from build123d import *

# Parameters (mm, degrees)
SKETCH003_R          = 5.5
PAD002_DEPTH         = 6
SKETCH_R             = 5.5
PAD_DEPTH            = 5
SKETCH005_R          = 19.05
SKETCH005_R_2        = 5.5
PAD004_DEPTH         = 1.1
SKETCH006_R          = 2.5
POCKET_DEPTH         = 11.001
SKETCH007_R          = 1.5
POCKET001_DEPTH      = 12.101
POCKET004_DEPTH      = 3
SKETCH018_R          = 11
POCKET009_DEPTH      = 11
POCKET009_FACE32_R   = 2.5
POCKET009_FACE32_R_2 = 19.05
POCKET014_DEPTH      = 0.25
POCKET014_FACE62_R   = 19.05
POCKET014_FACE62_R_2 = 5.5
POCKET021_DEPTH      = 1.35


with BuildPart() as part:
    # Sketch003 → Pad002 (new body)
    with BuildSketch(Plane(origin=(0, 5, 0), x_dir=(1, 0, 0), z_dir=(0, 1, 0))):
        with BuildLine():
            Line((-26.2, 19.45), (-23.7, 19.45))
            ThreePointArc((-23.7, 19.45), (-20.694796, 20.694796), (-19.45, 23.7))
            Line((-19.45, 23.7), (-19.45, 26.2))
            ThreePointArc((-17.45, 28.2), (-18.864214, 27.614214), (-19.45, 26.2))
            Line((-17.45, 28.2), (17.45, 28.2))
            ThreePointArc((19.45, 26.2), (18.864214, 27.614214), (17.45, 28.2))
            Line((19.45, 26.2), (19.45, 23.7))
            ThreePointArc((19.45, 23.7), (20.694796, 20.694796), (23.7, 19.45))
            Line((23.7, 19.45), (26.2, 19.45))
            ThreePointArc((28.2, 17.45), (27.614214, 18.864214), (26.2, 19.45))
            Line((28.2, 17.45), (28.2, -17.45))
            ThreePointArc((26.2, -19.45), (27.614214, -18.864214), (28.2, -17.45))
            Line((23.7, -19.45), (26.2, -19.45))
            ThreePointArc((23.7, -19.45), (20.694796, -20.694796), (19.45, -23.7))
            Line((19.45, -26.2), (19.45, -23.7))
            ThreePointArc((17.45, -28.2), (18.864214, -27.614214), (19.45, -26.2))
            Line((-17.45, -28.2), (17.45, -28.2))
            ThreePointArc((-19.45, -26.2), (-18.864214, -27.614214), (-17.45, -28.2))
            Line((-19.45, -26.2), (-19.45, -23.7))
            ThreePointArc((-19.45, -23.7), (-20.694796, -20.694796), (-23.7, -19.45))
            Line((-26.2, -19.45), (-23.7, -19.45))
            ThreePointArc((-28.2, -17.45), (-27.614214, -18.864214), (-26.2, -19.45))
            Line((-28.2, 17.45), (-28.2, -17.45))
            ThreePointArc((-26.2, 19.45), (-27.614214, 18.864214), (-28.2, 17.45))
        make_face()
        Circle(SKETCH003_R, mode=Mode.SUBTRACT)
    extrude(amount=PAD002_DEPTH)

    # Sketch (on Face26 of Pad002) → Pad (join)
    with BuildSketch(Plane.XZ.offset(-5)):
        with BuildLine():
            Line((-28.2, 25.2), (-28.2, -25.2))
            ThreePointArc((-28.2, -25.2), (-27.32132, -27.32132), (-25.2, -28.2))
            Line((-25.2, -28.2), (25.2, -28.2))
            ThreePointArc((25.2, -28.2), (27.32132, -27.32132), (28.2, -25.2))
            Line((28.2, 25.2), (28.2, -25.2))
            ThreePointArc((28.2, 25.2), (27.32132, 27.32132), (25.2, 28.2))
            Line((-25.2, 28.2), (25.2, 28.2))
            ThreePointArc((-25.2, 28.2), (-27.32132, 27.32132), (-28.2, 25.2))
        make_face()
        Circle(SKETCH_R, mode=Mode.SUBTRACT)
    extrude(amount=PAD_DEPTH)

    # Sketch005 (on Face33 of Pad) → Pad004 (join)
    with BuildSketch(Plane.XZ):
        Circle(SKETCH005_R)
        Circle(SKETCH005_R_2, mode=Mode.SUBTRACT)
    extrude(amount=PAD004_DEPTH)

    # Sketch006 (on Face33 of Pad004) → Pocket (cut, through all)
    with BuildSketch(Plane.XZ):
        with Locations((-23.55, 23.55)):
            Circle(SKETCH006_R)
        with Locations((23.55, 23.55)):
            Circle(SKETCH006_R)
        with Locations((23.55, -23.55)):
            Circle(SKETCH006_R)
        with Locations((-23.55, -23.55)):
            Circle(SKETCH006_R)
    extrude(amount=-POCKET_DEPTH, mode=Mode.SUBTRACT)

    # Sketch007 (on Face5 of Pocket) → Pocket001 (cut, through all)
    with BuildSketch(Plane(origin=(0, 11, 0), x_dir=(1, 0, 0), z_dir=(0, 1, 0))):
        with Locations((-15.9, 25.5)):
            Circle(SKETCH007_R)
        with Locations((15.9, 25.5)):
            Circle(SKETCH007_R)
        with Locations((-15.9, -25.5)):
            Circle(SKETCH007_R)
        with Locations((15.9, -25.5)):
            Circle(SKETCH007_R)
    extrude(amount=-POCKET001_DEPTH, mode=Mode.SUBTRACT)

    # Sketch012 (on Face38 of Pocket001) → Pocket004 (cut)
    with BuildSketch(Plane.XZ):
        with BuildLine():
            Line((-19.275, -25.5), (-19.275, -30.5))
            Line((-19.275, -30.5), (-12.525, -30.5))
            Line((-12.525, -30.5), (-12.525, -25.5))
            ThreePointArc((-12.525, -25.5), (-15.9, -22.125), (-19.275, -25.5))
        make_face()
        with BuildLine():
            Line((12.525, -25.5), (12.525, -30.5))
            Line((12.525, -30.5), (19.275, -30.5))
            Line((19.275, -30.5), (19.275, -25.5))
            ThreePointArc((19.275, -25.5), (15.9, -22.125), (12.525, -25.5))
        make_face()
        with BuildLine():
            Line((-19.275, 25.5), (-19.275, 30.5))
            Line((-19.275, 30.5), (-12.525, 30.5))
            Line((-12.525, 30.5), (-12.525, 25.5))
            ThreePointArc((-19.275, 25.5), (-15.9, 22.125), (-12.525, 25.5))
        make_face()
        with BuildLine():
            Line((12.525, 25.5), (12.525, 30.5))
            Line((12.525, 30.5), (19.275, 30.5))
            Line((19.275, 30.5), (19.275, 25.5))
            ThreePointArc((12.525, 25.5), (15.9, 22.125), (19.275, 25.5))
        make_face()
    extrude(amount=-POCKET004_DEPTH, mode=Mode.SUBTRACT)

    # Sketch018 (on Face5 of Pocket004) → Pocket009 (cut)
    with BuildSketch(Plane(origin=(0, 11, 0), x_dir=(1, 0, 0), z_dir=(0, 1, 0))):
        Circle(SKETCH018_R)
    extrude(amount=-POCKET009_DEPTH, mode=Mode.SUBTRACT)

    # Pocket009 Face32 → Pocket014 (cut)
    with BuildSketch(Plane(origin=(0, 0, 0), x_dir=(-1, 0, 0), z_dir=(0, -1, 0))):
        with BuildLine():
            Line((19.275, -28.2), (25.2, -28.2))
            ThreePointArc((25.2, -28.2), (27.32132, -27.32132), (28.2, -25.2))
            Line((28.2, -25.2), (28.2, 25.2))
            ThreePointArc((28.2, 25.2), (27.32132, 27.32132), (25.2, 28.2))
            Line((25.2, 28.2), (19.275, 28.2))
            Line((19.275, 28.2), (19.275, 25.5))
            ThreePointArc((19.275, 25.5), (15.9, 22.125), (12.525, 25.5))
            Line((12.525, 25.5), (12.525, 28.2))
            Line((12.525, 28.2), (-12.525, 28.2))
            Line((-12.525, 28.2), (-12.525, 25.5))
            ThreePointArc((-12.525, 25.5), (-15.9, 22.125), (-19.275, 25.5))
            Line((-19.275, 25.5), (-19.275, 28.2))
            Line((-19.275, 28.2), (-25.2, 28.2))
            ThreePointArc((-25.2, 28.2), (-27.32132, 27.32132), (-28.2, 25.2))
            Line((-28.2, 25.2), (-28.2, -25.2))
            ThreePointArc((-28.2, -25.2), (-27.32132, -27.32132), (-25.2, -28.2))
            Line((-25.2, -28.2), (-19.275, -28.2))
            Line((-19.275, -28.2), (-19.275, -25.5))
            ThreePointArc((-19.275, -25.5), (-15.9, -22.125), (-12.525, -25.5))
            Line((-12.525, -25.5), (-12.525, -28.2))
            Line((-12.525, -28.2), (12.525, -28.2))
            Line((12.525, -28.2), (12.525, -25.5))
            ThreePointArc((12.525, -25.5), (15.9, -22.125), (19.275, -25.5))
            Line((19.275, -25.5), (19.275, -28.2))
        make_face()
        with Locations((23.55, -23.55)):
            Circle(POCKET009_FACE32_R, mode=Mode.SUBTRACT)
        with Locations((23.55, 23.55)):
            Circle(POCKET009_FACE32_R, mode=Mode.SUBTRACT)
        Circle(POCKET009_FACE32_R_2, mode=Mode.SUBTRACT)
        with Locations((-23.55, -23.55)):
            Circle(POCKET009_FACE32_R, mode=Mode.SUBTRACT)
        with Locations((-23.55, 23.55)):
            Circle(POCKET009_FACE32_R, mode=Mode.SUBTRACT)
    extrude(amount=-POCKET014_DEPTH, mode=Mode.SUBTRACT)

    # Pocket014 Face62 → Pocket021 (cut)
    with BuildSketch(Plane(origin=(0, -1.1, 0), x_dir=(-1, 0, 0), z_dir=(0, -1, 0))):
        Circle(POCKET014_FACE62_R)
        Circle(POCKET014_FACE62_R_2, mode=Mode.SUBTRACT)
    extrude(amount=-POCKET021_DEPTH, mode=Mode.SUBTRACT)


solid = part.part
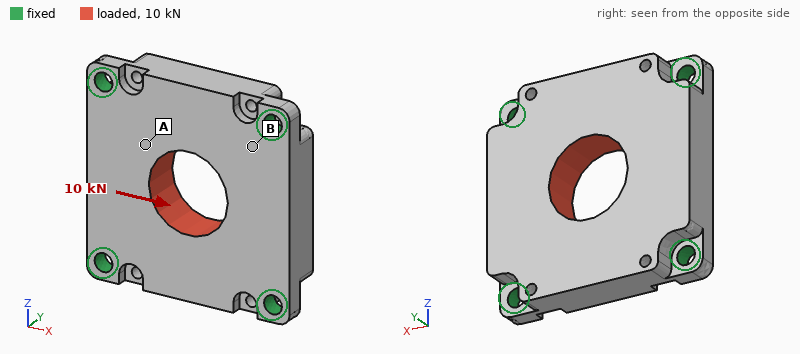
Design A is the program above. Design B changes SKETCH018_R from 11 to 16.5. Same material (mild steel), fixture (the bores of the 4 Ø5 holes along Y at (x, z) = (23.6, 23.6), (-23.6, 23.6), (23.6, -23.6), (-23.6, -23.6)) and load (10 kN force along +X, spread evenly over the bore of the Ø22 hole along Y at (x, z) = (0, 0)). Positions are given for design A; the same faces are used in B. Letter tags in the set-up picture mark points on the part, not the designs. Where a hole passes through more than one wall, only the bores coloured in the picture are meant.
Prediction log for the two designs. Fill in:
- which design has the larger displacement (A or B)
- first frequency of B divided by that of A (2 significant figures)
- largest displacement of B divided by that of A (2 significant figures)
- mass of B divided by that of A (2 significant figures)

B
1.1
1.3
0.81
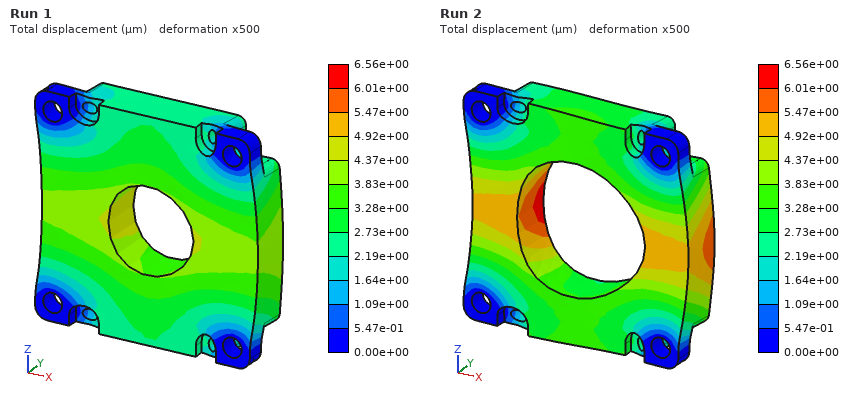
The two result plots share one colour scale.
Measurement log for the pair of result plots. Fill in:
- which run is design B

Run 2
